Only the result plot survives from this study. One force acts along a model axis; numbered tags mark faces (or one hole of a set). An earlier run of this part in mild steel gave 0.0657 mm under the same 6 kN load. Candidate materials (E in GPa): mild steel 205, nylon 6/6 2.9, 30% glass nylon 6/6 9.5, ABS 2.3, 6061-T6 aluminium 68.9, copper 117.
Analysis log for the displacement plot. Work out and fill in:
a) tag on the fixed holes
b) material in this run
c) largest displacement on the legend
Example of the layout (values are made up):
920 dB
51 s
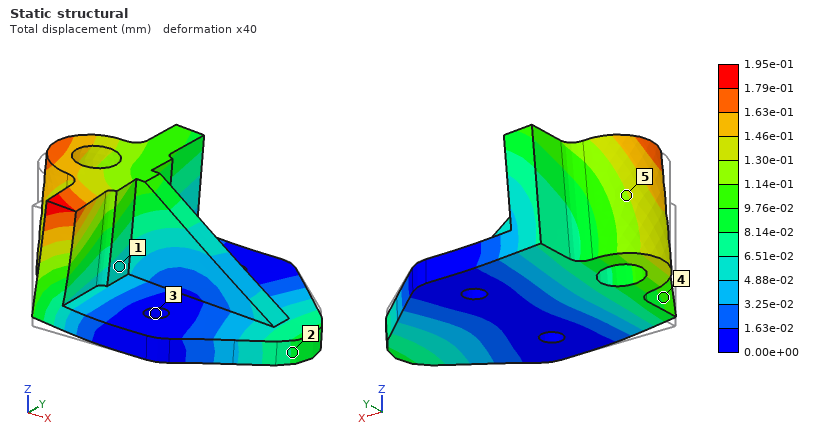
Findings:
3
6061-T6 aluminium
1.95e-01 mm
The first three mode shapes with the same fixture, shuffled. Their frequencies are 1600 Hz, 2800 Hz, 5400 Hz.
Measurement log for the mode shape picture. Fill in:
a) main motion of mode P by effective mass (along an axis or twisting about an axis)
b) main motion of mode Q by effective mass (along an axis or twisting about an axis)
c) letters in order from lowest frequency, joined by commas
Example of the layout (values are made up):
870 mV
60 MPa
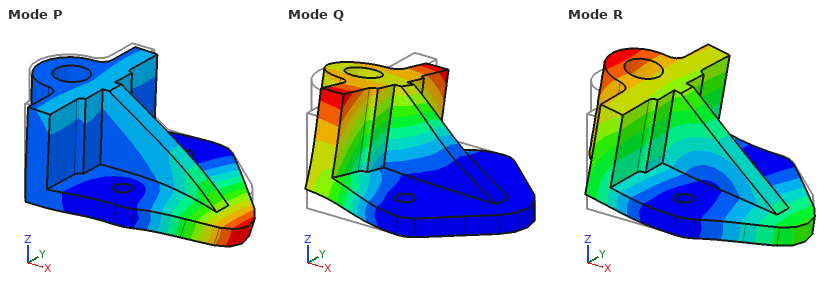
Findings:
along Z
along Y
R, Q, P
